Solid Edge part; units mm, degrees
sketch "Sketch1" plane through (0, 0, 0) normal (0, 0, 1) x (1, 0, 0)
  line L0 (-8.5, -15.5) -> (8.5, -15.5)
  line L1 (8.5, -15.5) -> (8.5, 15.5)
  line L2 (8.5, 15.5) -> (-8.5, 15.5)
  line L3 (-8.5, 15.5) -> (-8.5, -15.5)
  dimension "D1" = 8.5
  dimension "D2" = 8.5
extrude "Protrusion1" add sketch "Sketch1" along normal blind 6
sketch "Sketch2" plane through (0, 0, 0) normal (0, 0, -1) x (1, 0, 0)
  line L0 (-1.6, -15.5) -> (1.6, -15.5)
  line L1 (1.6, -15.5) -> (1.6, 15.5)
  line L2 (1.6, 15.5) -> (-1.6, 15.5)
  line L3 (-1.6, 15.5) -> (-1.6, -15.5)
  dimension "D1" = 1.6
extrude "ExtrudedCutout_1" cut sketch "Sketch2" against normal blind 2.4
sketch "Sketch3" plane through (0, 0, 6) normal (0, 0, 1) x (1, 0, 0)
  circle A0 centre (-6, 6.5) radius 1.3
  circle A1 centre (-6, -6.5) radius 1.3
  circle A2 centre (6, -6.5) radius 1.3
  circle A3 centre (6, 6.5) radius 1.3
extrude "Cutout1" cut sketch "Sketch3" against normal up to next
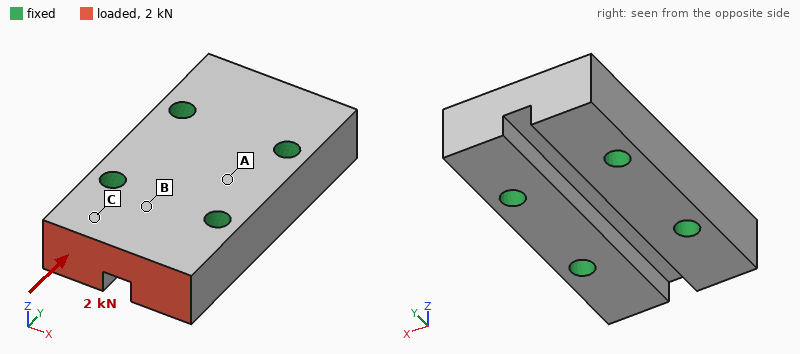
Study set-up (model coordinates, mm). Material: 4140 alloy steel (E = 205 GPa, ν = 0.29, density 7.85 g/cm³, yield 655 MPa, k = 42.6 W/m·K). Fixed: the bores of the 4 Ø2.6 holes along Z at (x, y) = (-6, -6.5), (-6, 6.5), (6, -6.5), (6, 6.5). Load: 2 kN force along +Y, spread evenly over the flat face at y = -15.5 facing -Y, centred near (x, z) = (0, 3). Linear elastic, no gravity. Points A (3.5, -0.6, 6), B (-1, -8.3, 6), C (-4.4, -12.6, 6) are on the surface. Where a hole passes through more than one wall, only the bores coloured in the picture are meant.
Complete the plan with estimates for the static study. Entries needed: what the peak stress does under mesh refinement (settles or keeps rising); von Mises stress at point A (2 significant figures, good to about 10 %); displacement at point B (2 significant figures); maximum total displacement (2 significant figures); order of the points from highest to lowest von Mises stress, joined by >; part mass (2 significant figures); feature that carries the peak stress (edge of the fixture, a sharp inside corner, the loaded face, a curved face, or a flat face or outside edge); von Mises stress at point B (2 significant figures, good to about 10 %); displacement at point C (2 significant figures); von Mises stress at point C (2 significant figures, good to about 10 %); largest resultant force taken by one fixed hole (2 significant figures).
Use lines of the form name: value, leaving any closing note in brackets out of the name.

what the peak stress does under mesh refinement: keeps rising
von Mises stress at point A: 4.5 MPa
displacement at point B: 0.48 µm
maximum total displacement: 1.1 µm
order of the points from highest to lowest von Mises stress, joined by >: C > B > A
part mass: 22 g
feature that carries the peak stress: edge of the fixture
von Mises stress at point B: 12 MPa
displacement at point C: 0.71 µm
von Mises stress at point C: 22 MPa
largest resultant force taken by one fixed hole: 930 N
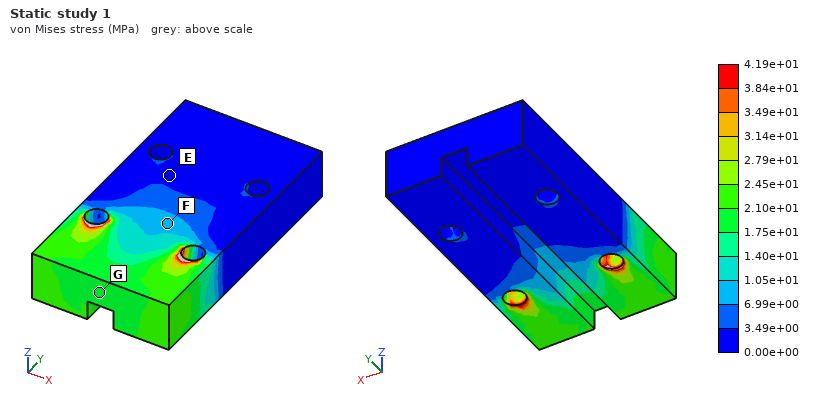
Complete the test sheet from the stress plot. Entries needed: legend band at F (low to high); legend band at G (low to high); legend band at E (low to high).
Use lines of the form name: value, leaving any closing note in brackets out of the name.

legend band at F: 6.99e+00 to 1.05e+01 MPa
legend band at G: 1.75e+01 to 2.10e+01 MPa
legend band at E: 0.00e+00 to 3.49e+00 MPa
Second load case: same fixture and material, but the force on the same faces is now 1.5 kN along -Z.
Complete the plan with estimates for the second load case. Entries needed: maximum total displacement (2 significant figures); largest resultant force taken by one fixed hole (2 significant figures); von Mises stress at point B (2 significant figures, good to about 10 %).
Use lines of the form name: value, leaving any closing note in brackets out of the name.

maximum total displacement: 9.5 µm
largest resultant force taken by one fixed hole: 820 N
von Mises stress at point B: 64 MPa
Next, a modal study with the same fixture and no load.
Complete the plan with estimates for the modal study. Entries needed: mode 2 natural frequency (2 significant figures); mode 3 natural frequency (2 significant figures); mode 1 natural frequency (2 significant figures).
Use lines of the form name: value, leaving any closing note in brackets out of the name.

mode 2 natural frequency: 48 kHz
mode 3 natural frequency: 62 kHz
mode 1 natural frequency: 48 kHz
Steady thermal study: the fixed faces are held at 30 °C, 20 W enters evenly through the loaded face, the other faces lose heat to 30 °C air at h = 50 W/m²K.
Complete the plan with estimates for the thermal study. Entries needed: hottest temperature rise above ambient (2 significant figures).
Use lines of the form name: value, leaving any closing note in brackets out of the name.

hottest temperature rise above ambient: 44 K
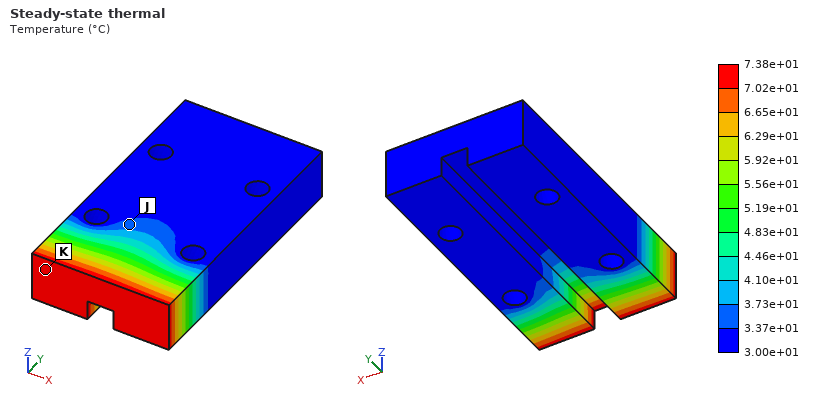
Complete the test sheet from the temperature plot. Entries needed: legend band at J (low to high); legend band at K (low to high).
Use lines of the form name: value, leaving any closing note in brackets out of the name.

legend band at J: 3.37e+01 to 3.73e+01 °C
legend band at K: 7.02e+01 to 7.38e+01 °C
